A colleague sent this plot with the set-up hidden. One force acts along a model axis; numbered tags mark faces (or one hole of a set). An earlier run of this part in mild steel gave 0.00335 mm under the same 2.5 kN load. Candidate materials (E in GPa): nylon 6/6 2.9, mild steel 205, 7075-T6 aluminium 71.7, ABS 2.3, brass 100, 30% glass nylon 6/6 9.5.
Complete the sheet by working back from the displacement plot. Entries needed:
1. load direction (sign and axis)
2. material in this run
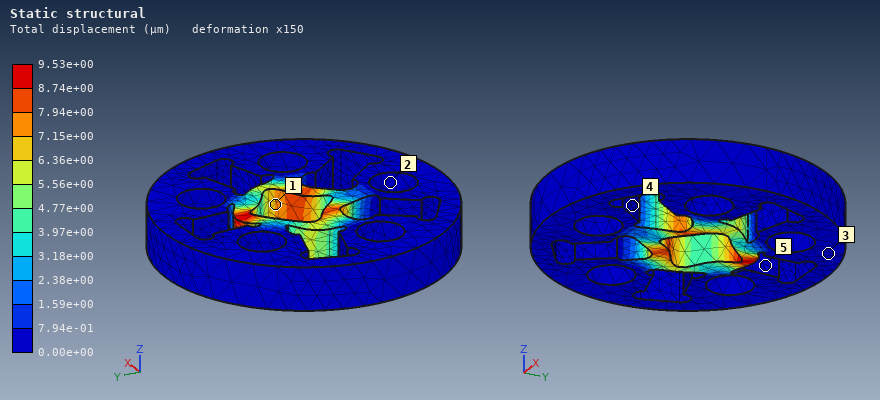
+Y
7075-T6 aluminium
